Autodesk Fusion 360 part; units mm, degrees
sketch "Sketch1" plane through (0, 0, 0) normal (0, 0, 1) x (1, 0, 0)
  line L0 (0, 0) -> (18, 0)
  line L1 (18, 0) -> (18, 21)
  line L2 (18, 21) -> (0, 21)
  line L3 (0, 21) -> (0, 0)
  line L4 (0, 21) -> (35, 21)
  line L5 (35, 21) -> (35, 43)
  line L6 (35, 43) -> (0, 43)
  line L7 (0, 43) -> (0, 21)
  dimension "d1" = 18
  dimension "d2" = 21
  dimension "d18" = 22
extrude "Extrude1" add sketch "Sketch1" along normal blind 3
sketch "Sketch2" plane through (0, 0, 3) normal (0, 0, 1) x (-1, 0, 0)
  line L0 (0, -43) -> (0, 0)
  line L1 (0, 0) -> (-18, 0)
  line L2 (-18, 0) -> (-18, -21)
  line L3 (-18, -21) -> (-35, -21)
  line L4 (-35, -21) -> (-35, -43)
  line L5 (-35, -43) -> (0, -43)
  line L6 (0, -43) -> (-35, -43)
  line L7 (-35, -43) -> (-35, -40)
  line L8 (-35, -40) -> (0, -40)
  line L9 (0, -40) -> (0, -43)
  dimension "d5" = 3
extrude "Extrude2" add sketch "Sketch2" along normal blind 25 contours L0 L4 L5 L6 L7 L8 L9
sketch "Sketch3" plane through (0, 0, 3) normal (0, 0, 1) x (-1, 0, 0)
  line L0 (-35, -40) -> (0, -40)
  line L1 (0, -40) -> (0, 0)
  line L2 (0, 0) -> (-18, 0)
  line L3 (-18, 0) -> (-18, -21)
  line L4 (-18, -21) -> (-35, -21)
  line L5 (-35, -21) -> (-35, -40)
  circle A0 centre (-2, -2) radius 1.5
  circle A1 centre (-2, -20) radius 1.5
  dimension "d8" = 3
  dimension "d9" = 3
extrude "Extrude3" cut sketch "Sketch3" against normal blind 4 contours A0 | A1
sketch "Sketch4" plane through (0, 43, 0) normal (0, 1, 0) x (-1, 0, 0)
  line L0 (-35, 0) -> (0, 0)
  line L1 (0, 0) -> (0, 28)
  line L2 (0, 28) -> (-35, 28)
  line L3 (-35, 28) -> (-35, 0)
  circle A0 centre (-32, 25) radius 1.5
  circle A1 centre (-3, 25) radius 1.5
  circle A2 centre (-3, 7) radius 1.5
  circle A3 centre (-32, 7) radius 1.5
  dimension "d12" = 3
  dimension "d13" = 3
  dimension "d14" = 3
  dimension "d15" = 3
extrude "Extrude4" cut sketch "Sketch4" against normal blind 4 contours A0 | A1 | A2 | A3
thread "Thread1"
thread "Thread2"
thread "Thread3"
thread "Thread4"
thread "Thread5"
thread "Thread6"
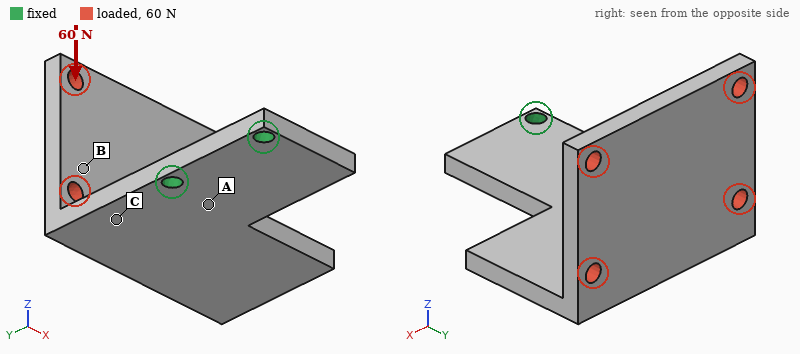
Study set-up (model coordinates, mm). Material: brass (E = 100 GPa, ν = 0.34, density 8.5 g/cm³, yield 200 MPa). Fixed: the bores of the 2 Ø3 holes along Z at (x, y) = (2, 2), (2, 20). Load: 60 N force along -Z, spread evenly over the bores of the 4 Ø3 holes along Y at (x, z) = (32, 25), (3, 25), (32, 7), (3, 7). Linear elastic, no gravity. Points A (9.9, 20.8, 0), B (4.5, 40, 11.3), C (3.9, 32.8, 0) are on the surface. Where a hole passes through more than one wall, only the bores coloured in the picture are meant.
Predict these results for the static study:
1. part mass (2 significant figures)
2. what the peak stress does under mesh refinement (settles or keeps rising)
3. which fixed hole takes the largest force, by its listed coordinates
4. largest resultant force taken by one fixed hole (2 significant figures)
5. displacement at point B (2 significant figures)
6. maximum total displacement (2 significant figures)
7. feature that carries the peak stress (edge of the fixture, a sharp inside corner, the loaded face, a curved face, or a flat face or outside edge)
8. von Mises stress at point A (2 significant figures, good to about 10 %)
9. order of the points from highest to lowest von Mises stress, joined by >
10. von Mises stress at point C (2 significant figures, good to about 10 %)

51 g
keeps rising
(2, 20)
97 N
0.063 mm
0.18 mm
edge of the fixture
37 MPa
A > C > B
20 MPa
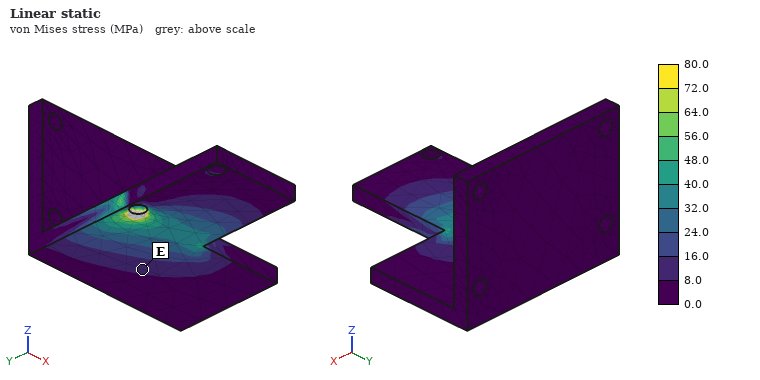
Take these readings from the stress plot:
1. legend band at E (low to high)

8.0 to 16.0 MPa
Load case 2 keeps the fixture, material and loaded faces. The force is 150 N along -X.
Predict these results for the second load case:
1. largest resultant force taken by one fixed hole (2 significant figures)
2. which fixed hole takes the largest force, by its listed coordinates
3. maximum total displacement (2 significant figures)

320 N
(2, 20)
0.30 mm
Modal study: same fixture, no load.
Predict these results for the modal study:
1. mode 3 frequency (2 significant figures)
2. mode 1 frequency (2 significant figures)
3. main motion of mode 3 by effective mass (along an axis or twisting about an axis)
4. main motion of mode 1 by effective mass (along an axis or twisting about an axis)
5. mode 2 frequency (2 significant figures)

2200 Hz
600 Hz
along Z
along Z
990 Hz
